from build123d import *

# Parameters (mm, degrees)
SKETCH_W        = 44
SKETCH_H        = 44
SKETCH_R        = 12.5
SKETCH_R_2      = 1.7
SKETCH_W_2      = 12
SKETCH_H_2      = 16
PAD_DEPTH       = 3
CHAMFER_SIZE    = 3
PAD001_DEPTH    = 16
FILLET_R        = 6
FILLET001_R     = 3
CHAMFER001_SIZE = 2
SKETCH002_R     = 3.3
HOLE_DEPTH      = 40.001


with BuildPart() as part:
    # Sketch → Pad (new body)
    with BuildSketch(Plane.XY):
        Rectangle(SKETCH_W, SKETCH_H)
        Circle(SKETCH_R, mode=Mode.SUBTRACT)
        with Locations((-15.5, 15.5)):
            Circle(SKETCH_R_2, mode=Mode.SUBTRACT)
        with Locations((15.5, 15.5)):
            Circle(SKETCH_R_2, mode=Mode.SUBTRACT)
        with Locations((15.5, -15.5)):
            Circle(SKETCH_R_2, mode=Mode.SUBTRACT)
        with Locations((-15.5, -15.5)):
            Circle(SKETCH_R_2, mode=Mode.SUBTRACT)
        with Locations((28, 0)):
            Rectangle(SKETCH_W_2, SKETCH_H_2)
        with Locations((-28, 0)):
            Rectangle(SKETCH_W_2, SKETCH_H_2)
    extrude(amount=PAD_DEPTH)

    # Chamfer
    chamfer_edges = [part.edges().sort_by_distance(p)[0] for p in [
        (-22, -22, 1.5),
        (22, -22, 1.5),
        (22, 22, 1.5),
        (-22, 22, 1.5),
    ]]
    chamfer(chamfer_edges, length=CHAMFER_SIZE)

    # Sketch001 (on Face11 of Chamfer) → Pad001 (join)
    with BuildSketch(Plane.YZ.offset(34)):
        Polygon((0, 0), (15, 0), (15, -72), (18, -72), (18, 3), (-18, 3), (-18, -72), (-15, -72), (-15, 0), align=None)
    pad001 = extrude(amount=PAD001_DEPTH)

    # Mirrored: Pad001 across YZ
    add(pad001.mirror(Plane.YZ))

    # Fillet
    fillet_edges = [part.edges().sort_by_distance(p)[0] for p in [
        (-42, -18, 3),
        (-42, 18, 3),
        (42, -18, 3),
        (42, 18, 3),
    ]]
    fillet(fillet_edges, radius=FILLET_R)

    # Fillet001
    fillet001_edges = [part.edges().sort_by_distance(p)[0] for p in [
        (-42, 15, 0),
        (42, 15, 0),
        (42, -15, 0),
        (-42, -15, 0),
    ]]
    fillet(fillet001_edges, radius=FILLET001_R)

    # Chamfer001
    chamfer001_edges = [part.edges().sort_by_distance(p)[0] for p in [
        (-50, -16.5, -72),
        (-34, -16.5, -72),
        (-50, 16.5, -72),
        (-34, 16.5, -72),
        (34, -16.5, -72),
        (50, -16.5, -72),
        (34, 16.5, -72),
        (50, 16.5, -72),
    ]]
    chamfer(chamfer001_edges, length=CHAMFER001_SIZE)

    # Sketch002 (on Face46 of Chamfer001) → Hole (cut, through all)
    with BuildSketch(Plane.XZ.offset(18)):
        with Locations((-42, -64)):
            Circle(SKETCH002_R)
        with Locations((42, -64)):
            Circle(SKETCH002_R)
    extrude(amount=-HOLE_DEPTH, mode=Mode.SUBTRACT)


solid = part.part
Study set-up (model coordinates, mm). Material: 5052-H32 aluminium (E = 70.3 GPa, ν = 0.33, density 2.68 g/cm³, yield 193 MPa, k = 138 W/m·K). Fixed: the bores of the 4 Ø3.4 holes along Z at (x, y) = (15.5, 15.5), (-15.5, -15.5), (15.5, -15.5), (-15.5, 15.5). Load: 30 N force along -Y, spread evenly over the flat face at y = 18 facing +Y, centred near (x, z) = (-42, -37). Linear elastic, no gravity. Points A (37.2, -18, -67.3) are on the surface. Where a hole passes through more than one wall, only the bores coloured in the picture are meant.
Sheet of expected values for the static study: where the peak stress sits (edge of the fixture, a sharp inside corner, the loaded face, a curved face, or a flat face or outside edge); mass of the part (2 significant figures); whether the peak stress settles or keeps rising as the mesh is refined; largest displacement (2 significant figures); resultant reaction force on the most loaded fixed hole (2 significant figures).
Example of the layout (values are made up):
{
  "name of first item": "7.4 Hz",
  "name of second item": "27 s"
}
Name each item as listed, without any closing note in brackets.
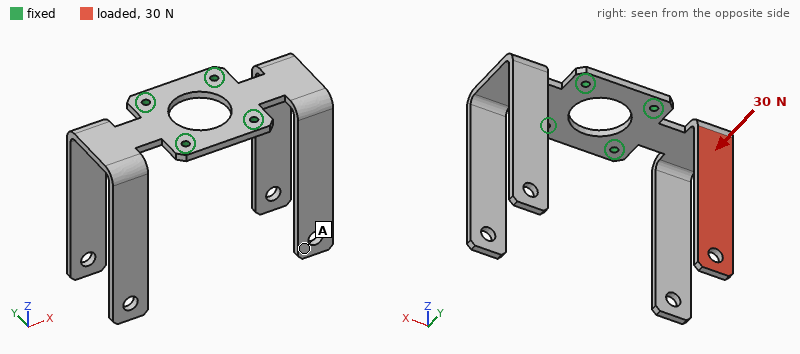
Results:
{
  "where the peak stress sits": "a sharp inside corner",
  "mass of the part": "58 g",
  "whether the peak stress settles or keeps rising as the mesh is refined": "keeps rising",
  "largest displacement": "1.4 mm",
  "resultant reaction force on the most loaded fixed hole": "62 N"
}
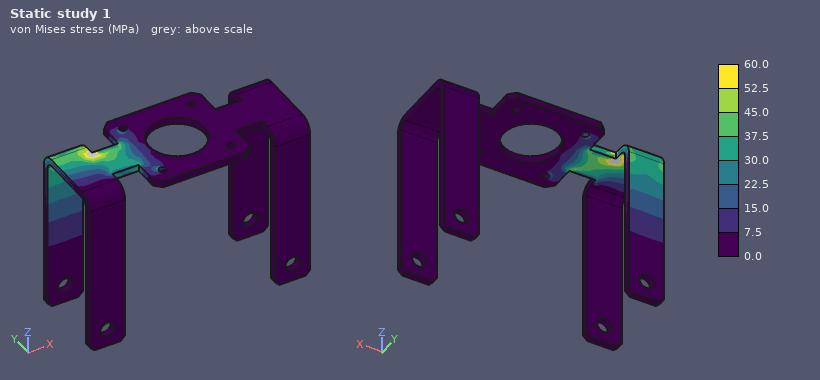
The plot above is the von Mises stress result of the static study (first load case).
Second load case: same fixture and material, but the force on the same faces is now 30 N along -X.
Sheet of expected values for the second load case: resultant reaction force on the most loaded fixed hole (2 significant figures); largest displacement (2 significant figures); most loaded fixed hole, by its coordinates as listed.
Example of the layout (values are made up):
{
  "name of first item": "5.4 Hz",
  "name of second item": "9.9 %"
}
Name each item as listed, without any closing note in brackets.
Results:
{
  "resultant reaction force on the most loaded fixed hole": "36 N",
  "largest displacement": "1.1 mm",
  "most loaded fixed hole, by its coordinates as listed": "(-15.5, 15.5)"
}
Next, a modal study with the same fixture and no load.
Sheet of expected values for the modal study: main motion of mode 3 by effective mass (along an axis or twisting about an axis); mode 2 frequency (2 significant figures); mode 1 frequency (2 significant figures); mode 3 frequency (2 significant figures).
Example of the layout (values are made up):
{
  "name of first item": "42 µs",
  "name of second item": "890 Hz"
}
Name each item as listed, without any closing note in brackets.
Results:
{
  "main motion of mode 3 by effective mass": "along Y",
  "mode 2 frequency": "260 Hz",
  "mode 1 frequency": "260 Hz",
  "mode 3 frequency": "270 Hz"
}
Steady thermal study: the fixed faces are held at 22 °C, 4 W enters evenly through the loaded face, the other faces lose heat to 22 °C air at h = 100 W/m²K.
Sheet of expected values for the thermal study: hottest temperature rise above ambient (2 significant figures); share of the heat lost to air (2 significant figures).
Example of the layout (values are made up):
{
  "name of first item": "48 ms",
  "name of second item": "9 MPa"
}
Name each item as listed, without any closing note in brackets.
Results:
{
  "hottest temperature rise above ambient": "16 K",
  "share of the heat lost to air": "79 %"
}
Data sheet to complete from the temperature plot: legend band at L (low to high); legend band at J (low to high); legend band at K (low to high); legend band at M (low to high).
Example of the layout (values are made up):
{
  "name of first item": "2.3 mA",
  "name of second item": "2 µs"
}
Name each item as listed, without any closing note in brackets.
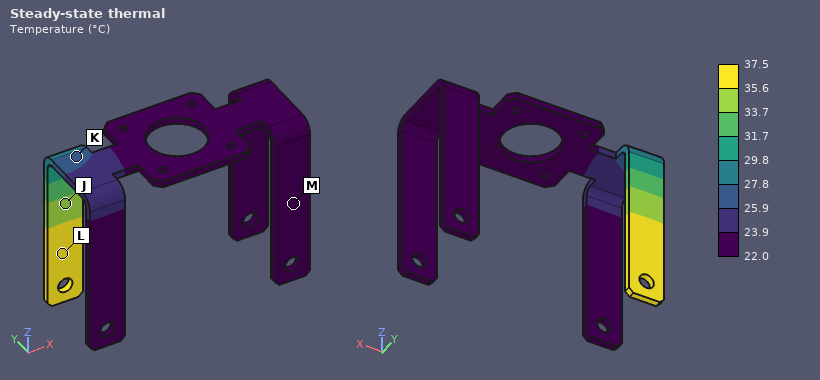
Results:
{
  "legend band at L": "35.6 to 37.5 °C",
  "legend band at J": "33.7 to 35.6 °C",
  "legend band at K": "25.9 to 27.8 °C",
  "legend band at M": "22.0 to 23.9 °C"
}
